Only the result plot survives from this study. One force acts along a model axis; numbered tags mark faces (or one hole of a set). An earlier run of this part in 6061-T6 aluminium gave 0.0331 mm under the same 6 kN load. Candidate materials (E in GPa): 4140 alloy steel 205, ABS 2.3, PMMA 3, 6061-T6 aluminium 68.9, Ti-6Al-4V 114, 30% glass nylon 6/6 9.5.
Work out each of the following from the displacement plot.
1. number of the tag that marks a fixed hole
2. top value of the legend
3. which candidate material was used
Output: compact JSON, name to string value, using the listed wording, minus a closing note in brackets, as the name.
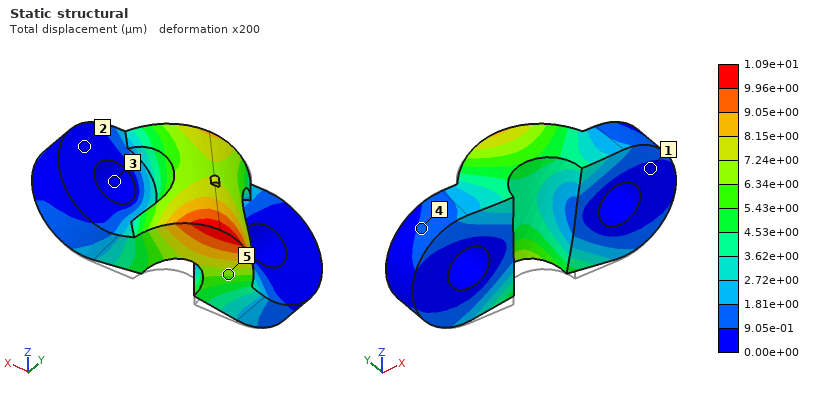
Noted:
{"number of the tag that marks a fixed hole": "3", "top value of the legend": "1.09e+01 µm", "which candidate material was used": "4140 alloy steel"}
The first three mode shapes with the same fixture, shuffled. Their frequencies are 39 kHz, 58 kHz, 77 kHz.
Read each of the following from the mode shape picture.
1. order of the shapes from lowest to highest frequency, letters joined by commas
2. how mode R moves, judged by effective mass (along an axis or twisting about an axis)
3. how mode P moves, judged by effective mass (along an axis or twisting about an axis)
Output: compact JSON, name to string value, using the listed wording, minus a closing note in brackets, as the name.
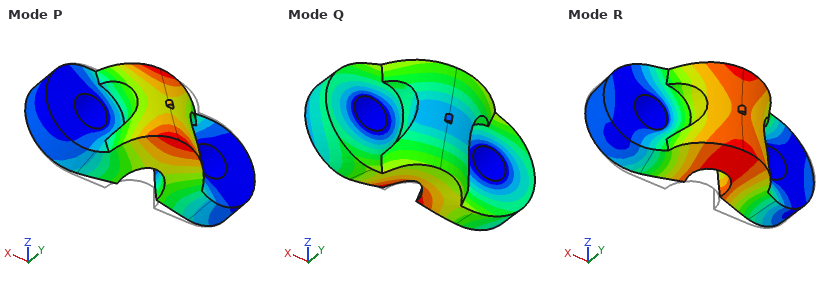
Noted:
{"order of the shapes from lowest to highest frequency, letters joined by commas": "P, R, Q", "how mode R moves, judged by effective mass": "along Y", "how mode P moves, judged by effective mass": "along Z"}
